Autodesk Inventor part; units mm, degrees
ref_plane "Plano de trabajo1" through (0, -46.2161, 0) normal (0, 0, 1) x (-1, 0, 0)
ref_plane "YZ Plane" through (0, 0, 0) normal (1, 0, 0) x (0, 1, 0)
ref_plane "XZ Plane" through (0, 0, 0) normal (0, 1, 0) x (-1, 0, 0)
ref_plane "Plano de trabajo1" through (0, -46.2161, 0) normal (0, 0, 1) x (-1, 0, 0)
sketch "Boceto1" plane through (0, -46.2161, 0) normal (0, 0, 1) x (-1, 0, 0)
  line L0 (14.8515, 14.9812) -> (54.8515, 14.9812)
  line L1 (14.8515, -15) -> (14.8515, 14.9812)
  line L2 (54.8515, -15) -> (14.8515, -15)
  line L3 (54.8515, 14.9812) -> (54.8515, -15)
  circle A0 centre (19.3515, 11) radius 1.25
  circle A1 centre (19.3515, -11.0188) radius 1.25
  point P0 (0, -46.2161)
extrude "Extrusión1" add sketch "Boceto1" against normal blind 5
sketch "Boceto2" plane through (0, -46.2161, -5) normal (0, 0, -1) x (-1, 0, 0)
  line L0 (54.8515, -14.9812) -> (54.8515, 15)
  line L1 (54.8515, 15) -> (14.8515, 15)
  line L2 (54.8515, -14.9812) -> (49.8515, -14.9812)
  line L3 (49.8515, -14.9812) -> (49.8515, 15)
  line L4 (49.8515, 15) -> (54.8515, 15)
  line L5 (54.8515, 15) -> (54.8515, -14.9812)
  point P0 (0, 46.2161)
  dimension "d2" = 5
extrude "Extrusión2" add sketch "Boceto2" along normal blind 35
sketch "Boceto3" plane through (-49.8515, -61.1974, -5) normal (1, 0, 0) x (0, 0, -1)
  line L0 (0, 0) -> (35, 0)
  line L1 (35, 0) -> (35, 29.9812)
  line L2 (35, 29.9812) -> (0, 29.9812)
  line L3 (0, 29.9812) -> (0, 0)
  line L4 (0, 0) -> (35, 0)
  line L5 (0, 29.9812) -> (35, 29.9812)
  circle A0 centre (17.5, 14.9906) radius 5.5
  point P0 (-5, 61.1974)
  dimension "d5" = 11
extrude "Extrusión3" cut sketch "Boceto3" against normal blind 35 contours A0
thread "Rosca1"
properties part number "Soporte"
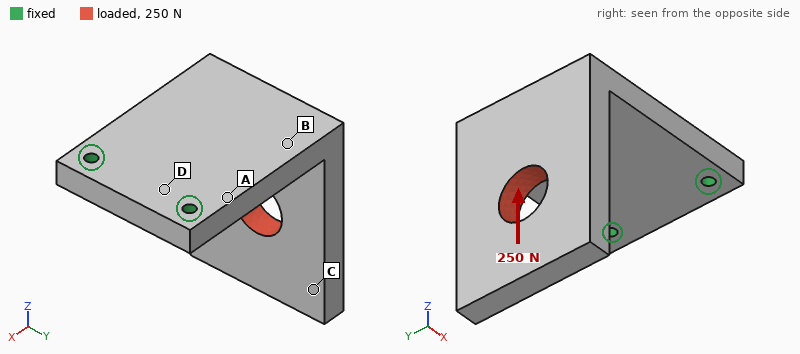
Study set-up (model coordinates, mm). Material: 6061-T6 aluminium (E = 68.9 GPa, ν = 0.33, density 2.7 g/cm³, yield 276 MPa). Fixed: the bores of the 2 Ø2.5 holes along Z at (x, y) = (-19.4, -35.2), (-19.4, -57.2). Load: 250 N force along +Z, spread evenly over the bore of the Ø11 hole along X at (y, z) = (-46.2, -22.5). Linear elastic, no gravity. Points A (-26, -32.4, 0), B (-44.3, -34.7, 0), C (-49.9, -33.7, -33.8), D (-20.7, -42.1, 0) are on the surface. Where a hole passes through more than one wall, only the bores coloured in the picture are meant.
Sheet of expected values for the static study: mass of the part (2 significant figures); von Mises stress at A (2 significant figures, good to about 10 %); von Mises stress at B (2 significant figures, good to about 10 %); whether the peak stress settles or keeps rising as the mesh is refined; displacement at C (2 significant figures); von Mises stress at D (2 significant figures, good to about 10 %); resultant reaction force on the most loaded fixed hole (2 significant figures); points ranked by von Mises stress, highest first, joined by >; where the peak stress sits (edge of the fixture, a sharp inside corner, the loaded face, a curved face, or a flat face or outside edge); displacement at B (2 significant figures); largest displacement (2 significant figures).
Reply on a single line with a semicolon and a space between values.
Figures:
29 g; 61 MPa; 18 MPa; keeps rising; 0.27 mm; 32 MPa; 130 N; A > D > B > C; edge of the fixture; 0.11 mm; 0.32 mm
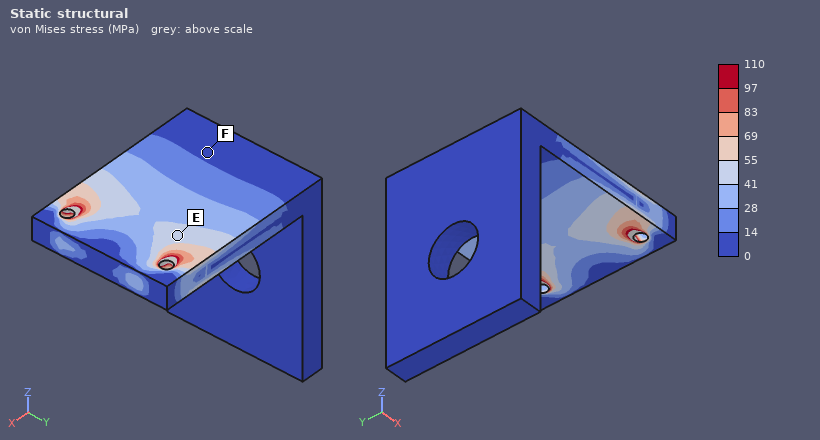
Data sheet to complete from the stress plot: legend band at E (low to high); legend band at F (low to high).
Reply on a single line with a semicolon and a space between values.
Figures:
41 to 55 MPa; 0 to 14 MPa
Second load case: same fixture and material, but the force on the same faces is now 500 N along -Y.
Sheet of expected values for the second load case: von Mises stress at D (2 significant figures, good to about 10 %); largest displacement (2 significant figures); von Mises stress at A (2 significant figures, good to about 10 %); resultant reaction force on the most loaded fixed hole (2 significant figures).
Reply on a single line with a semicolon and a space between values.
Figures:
22 MPa; 0.33 mm; 61 MPa; 870 N
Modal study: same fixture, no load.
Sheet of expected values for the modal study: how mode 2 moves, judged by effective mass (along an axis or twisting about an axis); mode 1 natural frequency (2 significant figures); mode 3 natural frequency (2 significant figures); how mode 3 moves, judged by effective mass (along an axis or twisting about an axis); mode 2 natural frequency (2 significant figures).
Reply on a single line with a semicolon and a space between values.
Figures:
along Y; 1100 Hz; 3000 Hz; along Z; 2000 Hz
